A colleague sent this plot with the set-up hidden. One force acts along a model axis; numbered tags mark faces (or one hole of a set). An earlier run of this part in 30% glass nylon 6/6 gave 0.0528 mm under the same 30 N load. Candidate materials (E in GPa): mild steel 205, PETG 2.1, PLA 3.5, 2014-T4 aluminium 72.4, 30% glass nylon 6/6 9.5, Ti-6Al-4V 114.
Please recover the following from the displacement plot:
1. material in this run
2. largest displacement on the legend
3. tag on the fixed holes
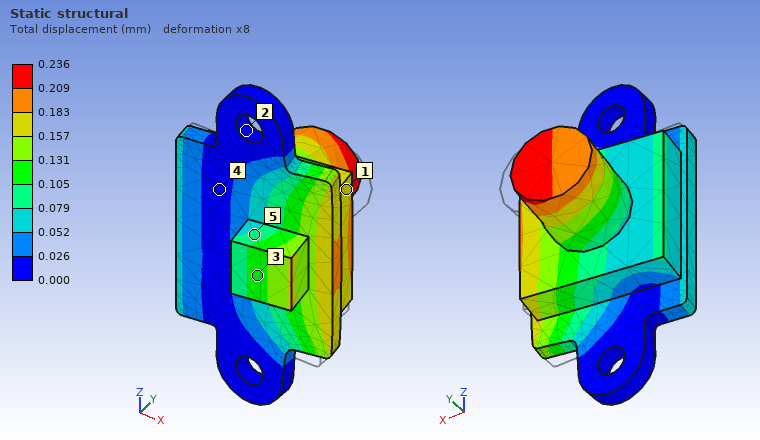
PETG
0.236 mm
2
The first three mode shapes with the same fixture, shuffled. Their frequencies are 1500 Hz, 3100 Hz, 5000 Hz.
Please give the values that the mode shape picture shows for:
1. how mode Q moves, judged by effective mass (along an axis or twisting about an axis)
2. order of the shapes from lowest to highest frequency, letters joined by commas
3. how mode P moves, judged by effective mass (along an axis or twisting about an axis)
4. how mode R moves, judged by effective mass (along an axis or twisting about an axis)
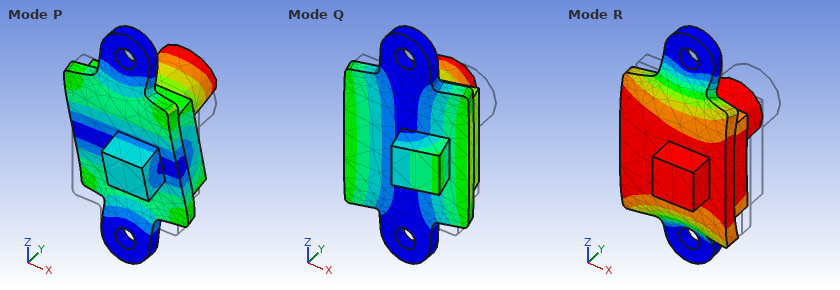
along X
Q, R, P
along Z
along Y
